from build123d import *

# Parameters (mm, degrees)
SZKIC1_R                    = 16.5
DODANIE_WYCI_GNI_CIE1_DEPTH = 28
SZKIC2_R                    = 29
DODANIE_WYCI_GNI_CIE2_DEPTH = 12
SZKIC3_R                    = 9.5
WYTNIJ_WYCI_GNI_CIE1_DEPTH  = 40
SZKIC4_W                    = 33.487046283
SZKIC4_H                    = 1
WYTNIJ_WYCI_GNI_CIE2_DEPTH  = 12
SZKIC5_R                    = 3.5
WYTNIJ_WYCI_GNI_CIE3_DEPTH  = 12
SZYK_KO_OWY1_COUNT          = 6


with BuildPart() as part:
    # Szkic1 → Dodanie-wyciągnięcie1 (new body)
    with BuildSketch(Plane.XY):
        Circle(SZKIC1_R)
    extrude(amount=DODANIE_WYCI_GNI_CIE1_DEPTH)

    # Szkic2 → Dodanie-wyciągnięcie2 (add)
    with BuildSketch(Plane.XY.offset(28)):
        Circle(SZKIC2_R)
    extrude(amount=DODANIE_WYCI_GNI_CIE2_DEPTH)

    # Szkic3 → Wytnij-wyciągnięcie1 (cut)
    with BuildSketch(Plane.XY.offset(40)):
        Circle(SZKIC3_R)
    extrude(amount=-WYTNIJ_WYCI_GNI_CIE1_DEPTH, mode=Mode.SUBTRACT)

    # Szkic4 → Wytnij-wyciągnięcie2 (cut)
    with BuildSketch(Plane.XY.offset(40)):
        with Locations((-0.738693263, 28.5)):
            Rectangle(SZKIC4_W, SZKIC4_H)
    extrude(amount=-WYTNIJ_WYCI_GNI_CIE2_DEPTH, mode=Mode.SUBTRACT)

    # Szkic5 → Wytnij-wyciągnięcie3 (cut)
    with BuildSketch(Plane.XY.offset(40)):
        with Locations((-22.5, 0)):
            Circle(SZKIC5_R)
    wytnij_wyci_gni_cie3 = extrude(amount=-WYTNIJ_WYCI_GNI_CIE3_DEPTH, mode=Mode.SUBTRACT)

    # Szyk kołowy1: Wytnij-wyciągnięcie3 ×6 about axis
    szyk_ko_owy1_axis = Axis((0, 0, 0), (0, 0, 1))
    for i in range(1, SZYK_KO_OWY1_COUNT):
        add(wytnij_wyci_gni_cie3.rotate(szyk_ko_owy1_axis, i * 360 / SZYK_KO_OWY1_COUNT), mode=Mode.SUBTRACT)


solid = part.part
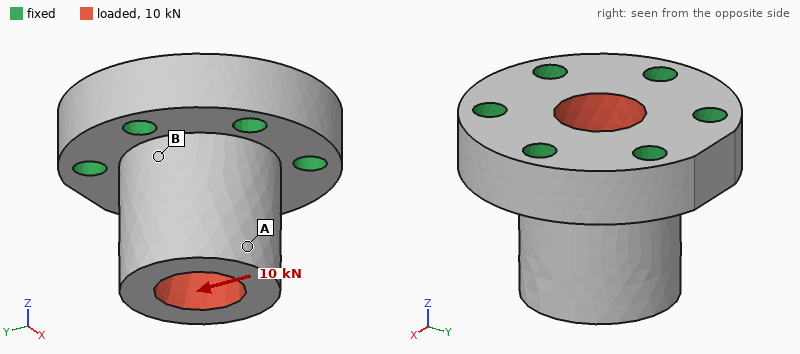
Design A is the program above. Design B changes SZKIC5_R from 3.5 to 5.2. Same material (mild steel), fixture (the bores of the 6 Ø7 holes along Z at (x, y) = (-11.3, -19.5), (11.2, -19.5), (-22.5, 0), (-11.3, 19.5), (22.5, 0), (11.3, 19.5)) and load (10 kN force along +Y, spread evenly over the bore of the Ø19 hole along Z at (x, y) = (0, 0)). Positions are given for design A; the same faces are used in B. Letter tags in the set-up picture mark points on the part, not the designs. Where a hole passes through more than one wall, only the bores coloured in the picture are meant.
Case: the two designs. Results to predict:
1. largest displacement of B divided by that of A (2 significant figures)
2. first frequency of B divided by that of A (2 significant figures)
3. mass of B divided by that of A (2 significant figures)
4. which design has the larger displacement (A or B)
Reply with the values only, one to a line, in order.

0.89
1.1
0.92
A
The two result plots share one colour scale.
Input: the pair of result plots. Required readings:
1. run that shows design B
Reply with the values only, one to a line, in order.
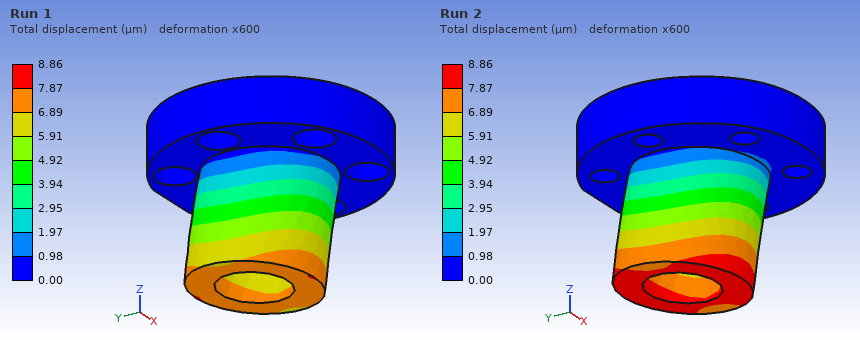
Run 1
